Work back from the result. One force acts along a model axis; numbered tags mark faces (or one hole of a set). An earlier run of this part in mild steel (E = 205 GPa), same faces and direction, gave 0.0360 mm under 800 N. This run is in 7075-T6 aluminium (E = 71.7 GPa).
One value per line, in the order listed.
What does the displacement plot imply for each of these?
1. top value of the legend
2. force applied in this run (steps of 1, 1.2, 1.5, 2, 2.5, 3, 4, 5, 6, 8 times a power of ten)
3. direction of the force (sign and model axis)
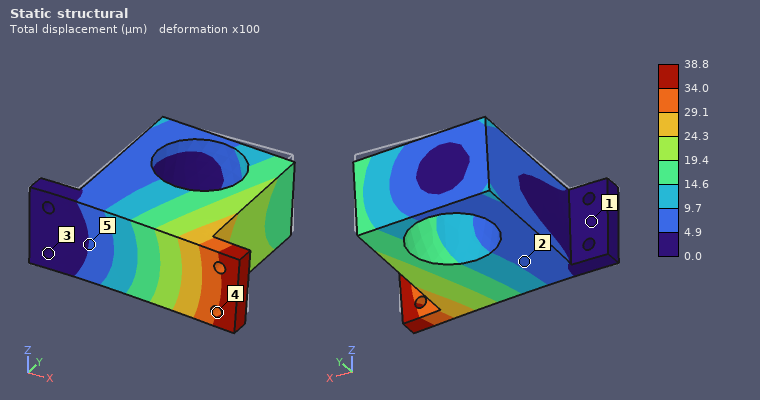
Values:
38.8 µm
300 N
-Z
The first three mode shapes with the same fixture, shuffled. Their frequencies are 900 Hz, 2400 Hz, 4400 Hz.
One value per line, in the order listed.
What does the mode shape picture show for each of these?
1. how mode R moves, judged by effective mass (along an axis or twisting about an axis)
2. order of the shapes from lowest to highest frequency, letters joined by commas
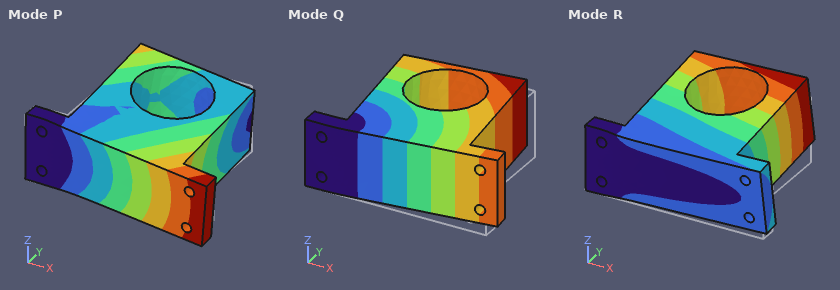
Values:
along Z
Q, R, P
